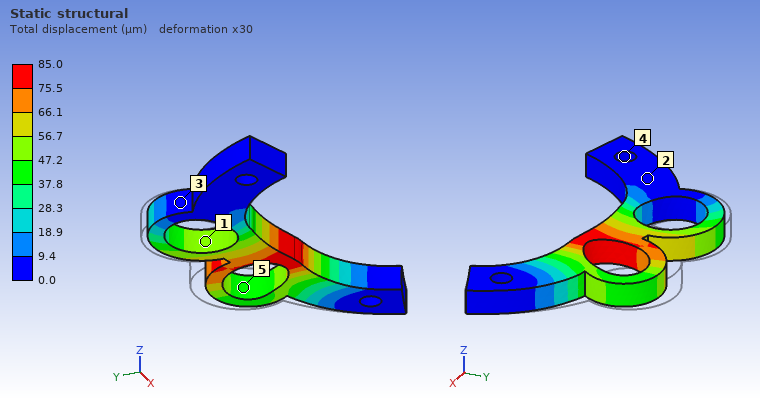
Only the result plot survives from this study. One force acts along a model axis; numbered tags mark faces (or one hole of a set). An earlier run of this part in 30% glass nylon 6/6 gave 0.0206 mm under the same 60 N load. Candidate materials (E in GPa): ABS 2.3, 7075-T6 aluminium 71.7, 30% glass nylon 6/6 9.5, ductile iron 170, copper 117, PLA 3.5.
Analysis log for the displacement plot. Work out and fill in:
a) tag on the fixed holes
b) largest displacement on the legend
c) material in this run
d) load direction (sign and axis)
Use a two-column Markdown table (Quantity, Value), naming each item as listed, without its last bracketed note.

| Quantity | Value |
|---|---|
| tag on the fixed holes | 4 |
| largest displacement on the legend | 85.0 µm |
| material in this run | ABS |
| load direction | -Y |
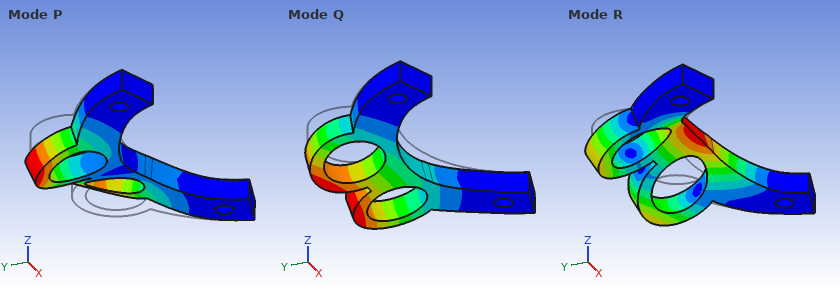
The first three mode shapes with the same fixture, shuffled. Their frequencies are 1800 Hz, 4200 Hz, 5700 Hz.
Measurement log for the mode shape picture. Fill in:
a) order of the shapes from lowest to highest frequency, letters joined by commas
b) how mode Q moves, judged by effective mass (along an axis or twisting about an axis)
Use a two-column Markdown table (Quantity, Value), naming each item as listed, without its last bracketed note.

| Quantity | Value |
|---|---|
| order of the shapes from lowest to highest frequency, letters joined by commas | Q, P, R |
| how mode Q moves, judged by effective mass | along Z |
